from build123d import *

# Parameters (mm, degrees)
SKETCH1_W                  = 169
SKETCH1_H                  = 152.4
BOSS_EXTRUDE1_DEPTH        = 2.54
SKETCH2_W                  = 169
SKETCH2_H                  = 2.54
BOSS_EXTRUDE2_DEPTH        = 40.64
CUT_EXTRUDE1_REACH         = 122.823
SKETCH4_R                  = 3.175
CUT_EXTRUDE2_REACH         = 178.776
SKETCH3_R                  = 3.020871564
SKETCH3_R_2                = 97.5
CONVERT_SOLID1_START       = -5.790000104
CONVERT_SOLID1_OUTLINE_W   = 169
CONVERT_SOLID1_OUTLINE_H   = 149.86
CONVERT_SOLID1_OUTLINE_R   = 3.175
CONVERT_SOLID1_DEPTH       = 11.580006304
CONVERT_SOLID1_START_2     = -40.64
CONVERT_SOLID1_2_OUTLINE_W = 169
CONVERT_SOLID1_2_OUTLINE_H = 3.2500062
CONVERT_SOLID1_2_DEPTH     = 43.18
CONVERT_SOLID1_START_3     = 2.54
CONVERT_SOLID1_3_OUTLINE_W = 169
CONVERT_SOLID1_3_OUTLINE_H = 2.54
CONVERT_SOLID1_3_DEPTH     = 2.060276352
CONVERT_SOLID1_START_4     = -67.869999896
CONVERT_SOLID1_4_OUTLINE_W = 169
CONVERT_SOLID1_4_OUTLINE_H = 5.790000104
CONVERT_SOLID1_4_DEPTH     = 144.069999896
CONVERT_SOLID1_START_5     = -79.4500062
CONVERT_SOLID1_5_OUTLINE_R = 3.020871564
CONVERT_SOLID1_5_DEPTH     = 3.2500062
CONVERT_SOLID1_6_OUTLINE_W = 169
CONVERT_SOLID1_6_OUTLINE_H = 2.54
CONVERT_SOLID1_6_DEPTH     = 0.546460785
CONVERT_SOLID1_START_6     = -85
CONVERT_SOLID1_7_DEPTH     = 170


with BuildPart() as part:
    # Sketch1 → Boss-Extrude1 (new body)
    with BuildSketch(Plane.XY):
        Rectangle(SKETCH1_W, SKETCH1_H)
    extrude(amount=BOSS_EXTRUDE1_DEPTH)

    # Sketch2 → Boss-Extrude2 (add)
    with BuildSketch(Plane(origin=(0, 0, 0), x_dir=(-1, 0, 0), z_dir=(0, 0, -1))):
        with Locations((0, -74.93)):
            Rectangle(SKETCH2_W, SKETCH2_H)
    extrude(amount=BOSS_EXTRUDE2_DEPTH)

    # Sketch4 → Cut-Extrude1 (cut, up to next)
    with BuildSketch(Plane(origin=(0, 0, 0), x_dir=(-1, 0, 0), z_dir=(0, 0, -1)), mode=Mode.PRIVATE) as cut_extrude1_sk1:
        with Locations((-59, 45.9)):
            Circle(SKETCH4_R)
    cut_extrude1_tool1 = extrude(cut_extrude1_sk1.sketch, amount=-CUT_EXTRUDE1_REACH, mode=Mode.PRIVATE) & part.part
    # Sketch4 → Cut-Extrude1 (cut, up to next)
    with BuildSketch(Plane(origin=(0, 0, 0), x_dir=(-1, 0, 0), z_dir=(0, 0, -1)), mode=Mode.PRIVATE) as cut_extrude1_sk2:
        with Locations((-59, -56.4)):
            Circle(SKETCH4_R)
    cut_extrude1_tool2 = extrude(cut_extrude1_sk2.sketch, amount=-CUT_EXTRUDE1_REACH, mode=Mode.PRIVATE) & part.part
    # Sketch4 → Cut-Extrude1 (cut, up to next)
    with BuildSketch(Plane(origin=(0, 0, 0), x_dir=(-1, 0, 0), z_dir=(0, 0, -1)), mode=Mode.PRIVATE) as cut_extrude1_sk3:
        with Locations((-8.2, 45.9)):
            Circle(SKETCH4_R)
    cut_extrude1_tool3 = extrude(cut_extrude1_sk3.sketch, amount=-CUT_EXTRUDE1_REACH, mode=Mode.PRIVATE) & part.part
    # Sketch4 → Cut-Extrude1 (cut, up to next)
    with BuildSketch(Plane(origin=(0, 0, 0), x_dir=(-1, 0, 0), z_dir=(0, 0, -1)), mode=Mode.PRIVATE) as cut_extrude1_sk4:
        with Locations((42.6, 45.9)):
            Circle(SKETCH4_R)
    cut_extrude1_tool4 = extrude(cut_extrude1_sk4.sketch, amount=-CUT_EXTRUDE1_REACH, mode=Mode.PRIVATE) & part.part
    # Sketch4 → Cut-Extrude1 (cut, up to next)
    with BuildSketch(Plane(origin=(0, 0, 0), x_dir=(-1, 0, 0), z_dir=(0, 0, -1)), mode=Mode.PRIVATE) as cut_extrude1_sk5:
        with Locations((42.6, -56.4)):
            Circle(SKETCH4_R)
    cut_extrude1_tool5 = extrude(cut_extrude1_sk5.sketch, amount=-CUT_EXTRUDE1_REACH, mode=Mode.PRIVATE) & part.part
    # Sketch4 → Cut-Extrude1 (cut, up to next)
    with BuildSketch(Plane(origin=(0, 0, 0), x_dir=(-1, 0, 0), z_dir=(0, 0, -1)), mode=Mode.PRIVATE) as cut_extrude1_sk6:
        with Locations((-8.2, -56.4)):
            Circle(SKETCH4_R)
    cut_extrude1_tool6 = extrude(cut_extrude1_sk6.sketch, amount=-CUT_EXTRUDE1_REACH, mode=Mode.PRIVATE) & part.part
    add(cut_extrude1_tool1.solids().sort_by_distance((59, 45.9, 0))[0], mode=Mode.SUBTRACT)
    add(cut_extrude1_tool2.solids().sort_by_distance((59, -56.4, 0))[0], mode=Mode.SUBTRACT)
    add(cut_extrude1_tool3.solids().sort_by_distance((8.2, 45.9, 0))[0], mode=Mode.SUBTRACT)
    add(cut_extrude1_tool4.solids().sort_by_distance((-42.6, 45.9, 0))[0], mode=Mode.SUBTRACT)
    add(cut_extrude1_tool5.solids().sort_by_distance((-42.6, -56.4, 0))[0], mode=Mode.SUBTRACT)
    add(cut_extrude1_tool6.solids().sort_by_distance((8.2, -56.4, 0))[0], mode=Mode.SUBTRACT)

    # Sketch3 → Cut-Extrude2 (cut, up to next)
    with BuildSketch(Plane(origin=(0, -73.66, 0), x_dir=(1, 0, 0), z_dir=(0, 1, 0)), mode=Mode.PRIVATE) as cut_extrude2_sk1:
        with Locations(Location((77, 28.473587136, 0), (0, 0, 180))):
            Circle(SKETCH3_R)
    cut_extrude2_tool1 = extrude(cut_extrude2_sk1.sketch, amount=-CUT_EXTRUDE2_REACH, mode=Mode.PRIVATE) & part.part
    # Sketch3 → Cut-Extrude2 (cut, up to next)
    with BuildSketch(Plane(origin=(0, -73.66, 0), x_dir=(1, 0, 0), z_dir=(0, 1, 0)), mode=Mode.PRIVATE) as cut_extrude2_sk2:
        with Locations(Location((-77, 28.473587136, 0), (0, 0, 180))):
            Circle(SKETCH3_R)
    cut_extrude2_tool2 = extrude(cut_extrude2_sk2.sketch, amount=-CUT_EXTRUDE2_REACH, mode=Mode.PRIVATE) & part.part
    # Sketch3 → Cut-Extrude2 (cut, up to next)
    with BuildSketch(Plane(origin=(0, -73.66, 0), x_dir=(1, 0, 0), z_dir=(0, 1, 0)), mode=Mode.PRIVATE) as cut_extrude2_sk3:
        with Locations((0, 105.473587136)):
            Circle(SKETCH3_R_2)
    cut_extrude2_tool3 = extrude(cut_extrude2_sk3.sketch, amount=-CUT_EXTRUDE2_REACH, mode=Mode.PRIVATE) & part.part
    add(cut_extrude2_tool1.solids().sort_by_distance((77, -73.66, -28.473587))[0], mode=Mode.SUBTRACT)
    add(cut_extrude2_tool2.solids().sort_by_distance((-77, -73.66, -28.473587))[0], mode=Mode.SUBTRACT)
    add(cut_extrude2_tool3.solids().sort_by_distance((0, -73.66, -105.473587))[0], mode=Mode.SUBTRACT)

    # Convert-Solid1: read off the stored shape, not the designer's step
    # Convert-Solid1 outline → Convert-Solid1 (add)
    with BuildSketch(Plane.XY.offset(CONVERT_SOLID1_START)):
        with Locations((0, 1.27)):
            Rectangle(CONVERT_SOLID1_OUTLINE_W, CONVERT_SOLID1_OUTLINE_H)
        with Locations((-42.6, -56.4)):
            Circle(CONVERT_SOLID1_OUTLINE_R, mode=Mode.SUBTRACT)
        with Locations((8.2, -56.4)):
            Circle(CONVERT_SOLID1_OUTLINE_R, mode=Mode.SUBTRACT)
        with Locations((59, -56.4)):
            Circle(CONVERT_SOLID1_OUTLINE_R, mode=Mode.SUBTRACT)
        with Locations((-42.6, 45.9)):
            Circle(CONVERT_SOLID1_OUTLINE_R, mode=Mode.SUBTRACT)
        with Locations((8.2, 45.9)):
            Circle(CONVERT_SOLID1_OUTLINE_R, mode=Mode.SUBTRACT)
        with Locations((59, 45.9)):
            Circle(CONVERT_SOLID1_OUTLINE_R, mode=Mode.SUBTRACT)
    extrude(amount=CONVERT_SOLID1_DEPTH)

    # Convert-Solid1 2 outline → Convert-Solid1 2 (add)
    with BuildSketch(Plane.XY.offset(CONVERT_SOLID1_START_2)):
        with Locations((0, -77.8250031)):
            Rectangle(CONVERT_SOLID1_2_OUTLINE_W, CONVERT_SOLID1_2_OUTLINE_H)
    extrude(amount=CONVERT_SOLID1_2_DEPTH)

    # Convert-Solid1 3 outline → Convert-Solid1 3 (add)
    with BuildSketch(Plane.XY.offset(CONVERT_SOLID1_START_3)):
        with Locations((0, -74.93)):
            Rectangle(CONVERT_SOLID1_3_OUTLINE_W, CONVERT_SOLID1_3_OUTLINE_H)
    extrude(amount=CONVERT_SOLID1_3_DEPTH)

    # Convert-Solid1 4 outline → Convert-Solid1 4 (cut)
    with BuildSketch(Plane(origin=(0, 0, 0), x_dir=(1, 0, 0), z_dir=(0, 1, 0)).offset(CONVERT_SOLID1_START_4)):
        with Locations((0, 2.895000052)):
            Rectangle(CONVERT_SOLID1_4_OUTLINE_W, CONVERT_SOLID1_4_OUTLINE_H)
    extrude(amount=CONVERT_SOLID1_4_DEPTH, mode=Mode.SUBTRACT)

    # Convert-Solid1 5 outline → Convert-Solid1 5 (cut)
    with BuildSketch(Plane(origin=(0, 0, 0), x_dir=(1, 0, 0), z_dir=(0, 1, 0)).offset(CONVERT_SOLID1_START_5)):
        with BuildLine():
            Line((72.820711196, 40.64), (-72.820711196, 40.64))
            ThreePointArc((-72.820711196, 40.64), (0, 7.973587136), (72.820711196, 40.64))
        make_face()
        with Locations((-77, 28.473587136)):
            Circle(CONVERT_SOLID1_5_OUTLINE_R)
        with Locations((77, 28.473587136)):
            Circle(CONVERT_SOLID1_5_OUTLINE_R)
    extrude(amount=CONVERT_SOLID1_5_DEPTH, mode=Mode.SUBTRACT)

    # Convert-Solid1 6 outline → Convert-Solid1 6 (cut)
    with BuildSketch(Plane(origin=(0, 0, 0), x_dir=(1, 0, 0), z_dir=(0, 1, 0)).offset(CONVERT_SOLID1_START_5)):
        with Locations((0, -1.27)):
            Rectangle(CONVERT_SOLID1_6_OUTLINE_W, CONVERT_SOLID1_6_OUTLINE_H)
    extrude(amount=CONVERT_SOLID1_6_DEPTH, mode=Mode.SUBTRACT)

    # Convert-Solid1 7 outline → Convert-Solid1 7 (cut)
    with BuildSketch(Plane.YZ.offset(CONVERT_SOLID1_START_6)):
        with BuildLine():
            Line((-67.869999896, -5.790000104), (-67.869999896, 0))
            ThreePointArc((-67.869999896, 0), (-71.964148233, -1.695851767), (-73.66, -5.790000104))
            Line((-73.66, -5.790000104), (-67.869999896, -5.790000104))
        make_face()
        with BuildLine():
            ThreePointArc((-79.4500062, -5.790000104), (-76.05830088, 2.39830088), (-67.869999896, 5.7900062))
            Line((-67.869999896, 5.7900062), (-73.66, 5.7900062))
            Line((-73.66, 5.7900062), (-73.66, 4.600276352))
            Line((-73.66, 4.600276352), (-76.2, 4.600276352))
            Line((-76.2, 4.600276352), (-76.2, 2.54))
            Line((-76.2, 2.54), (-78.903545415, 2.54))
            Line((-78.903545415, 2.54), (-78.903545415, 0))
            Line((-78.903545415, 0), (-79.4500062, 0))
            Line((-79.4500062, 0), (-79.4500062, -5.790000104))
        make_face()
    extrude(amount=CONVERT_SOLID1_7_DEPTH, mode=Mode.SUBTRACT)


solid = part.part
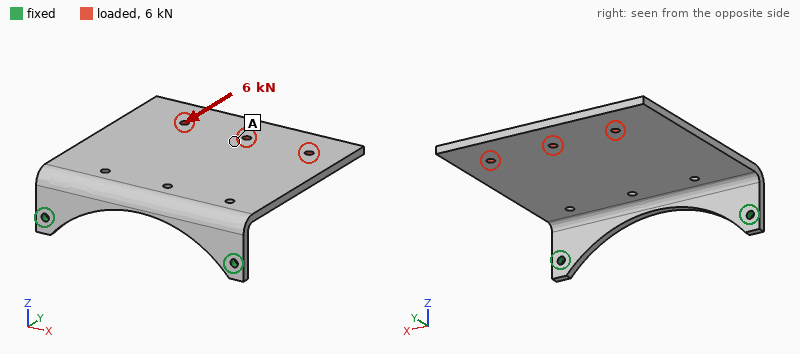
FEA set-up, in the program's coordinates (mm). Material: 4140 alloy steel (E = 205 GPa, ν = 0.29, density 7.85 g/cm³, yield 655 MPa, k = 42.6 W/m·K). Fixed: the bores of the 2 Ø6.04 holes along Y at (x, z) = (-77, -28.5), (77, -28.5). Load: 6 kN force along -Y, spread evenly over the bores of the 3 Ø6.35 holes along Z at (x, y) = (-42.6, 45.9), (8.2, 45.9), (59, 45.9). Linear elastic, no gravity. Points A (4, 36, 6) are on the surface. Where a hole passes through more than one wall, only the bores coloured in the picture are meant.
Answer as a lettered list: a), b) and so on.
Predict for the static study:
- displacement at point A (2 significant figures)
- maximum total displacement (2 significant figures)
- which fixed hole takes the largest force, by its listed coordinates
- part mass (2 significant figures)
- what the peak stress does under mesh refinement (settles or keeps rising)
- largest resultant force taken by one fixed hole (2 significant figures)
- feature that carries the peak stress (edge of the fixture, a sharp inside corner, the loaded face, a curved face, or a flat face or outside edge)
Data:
a) 1.7 mm
b) 2.3 mm
c) (77, -28.5)
d) 1.3 kg
e) keeps rising
f) 3.3 kN
g) edge of the fixture
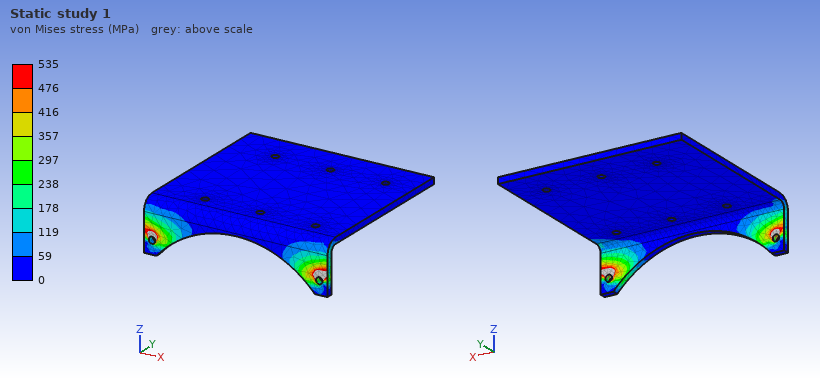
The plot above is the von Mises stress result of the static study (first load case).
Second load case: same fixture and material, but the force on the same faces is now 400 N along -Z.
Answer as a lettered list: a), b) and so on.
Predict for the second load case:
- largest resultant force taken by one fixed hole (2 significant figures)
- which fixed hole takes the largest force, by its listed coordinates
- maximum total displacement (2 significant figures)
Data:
a) 270 N
b) (77, -28.5)
c) 1.7 mm
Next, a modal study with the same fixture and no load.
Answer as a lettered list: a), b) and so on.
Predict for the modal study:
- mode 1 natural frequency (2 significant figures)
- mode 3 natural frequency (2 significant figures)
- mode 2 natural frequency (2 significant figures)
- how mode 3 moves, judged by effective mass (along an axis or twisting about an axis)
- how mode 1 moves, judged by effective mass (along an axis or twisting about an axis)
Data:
a) 120 Hz
b) 670 Hz
c) 390 Hz
d) along X
e) along Z
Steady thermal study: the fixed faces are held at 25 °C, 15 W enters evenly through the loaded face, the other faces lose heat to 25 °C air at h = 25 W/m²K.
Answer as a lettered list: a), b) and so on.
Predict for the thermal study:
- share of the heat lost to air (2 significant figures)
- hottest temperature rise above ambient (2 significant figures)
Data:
a) 92 %
b) 22 K
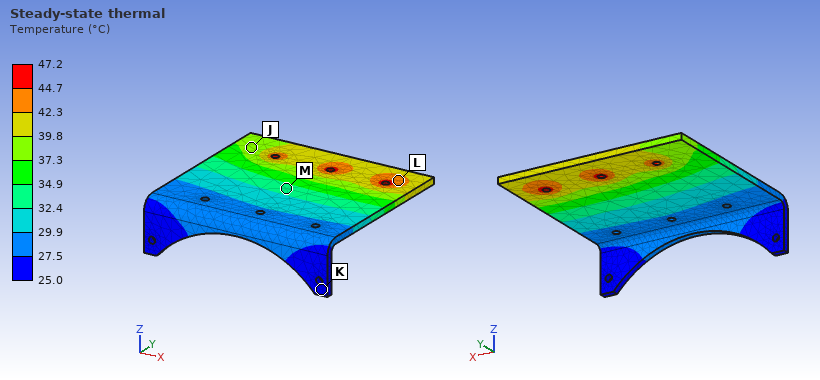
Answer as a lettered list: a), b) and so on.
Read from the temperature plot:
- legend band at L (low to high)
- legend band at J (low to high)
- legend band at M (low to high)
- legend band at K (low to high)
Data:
a) 42.3 to 44.7 °C
b) 37.3 to 39.8 °C
c) 32.4 to 34.9 °C
d) 25.0 to 27.5 °C
